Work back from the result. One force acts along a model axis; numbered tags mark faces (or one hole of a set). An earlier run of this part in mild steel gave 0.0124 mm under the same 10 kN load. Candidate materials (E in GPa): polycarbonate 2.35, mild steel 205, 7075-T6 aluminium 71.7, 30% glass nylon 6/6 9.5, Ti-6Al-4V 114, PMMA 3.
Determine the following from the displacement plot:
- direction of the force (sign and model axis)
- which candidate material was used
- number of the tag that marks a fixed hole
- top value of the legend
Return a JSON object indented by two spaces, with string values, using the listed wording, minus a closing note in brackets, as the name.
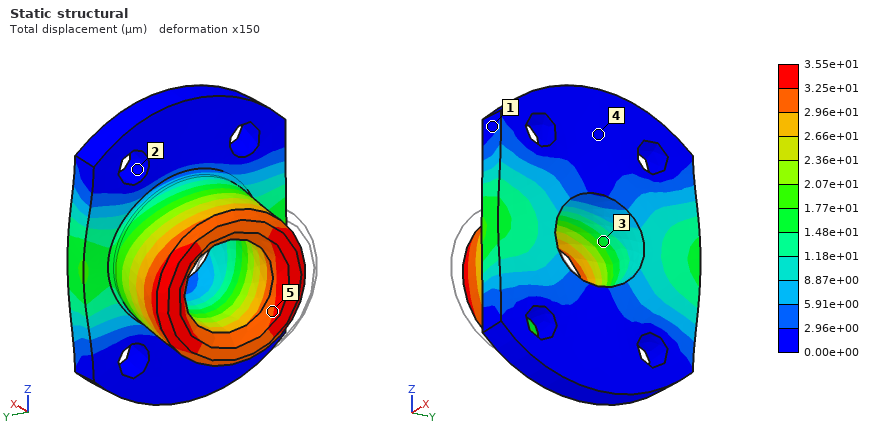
{
  "direction of the force": "+Y",
  "which candidate material was used": "7075-T6 aluminium",
  "number of the tag that marks a fixed hole": "2",
  "top value of the legend": "3.55e+01 µm"
}
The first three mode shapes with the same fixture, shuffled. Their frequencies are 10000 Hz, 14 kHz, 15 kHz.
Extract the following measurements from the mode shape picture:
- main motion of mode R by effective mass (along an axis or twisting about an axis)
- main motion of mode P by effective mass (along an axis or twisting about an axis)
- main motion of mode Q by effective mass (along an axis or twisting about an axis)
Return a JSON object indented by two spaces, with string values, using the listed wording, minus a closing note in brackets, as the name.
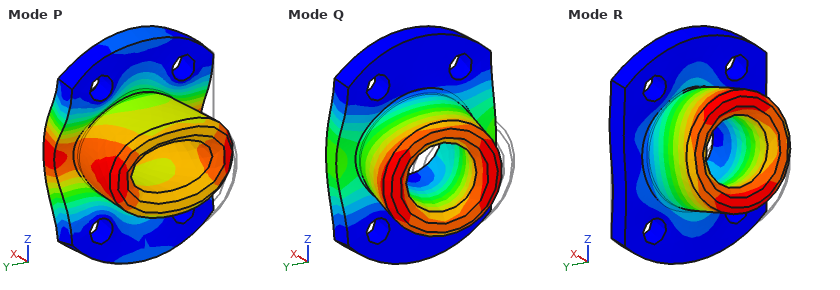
{
  "main motion of mode R by effective mass": "along Z",
  "main motion of mode P by effective mass": "along X",
  "main motion of mode Q by effective mass": "along Y"
}
